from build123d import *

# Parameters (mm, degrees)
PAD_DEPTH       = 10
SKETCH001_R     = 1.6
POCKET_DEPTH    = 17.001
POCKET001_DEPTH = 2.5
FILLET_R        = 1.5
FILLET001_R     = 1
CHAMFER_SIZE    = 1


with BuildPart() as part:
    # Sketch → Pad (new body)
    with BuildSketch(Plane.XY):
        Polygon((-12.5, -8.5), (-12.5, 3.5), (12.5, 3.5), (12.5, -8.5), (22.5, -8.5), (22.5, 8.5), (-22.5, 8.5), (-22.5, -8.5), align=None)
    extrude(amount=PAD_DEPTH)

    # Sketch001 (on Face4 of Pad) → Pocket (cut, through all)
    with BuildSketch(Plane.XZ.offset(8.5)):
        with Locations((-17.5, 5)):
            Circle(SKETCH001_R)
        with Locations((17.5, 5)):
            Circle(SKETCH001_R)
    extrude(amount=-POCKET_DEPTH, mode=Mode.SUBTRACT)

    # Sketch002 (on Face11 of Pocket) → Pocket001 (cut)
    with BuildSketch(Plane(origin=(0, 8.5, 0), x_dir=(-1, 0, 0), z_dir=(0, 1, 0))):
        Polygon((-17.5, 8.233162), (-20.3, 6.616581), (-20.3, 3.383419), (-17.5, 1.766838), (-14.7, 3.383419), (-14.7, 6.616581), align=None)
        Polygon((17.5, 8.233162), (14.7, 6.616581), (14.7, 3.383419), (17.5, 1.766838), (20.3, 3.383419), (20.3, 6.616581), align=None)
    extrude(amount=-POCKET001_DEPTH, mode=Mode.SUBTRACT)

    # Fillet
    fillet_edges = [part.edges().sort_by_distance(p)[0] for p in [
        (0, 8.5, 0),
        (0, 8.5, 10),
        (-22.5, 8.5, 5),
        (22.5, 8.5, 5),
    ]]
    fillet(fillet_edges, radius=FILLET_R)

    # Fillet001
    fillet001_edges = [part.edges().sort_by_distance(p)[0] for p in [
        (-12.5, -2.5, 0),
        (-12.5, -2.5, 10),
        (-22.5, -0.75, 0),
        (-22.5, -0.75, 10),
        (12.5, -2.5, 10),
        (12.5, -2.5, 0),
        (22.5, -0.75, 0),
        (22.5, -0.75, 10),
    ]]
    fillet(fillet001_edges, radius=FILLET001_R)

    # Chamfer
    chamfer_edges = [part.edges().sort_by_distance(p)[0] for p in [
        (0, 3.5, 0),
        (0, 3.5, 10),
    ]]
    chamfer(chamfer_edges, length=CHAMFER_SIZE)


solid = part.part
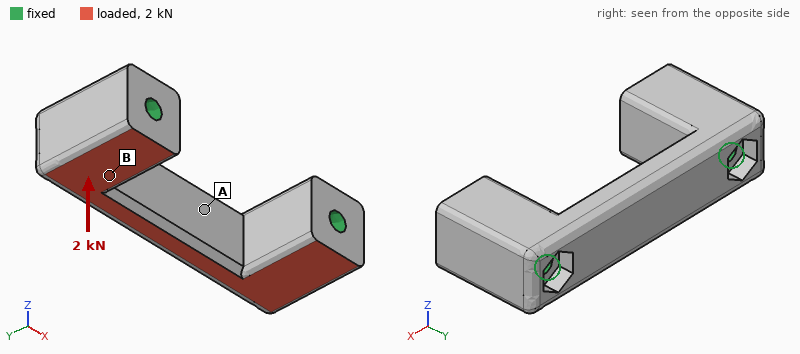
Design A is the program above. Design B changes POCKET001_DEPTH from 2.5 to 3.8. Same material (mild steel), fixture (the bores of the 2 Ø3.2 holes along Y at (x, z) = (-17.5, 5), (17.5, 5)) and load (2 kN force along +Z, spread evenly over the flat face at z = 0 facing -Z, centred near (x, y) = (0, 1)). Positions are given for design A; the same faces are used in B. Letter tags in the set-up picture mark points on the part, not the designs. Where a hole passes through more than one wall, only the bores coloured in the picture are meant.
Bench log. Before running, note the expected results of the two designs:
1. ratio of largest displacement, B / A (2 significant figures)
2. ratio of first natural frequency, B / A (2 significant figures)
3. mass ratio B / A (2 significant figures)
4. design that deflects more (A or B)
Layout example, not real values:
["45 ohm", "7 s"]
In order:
["1.2", "0.99", "0.99", "B"]
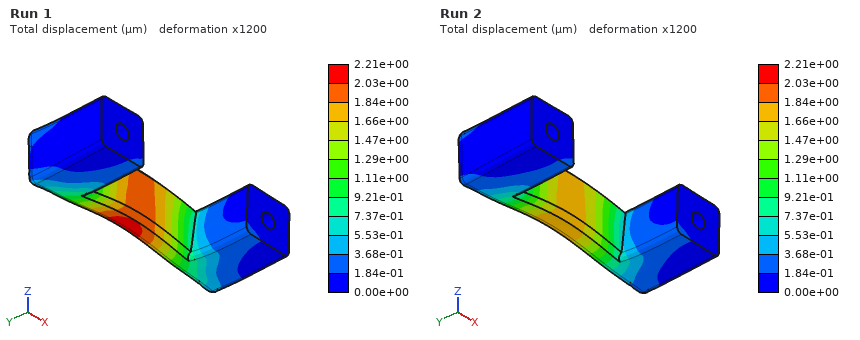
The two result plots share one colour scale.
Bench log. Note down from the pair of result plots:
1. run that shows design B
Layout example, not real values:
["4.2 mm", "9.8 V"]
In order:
["Run 1"]
